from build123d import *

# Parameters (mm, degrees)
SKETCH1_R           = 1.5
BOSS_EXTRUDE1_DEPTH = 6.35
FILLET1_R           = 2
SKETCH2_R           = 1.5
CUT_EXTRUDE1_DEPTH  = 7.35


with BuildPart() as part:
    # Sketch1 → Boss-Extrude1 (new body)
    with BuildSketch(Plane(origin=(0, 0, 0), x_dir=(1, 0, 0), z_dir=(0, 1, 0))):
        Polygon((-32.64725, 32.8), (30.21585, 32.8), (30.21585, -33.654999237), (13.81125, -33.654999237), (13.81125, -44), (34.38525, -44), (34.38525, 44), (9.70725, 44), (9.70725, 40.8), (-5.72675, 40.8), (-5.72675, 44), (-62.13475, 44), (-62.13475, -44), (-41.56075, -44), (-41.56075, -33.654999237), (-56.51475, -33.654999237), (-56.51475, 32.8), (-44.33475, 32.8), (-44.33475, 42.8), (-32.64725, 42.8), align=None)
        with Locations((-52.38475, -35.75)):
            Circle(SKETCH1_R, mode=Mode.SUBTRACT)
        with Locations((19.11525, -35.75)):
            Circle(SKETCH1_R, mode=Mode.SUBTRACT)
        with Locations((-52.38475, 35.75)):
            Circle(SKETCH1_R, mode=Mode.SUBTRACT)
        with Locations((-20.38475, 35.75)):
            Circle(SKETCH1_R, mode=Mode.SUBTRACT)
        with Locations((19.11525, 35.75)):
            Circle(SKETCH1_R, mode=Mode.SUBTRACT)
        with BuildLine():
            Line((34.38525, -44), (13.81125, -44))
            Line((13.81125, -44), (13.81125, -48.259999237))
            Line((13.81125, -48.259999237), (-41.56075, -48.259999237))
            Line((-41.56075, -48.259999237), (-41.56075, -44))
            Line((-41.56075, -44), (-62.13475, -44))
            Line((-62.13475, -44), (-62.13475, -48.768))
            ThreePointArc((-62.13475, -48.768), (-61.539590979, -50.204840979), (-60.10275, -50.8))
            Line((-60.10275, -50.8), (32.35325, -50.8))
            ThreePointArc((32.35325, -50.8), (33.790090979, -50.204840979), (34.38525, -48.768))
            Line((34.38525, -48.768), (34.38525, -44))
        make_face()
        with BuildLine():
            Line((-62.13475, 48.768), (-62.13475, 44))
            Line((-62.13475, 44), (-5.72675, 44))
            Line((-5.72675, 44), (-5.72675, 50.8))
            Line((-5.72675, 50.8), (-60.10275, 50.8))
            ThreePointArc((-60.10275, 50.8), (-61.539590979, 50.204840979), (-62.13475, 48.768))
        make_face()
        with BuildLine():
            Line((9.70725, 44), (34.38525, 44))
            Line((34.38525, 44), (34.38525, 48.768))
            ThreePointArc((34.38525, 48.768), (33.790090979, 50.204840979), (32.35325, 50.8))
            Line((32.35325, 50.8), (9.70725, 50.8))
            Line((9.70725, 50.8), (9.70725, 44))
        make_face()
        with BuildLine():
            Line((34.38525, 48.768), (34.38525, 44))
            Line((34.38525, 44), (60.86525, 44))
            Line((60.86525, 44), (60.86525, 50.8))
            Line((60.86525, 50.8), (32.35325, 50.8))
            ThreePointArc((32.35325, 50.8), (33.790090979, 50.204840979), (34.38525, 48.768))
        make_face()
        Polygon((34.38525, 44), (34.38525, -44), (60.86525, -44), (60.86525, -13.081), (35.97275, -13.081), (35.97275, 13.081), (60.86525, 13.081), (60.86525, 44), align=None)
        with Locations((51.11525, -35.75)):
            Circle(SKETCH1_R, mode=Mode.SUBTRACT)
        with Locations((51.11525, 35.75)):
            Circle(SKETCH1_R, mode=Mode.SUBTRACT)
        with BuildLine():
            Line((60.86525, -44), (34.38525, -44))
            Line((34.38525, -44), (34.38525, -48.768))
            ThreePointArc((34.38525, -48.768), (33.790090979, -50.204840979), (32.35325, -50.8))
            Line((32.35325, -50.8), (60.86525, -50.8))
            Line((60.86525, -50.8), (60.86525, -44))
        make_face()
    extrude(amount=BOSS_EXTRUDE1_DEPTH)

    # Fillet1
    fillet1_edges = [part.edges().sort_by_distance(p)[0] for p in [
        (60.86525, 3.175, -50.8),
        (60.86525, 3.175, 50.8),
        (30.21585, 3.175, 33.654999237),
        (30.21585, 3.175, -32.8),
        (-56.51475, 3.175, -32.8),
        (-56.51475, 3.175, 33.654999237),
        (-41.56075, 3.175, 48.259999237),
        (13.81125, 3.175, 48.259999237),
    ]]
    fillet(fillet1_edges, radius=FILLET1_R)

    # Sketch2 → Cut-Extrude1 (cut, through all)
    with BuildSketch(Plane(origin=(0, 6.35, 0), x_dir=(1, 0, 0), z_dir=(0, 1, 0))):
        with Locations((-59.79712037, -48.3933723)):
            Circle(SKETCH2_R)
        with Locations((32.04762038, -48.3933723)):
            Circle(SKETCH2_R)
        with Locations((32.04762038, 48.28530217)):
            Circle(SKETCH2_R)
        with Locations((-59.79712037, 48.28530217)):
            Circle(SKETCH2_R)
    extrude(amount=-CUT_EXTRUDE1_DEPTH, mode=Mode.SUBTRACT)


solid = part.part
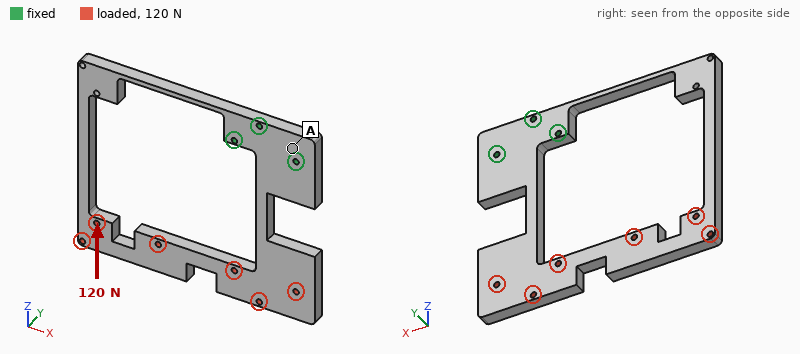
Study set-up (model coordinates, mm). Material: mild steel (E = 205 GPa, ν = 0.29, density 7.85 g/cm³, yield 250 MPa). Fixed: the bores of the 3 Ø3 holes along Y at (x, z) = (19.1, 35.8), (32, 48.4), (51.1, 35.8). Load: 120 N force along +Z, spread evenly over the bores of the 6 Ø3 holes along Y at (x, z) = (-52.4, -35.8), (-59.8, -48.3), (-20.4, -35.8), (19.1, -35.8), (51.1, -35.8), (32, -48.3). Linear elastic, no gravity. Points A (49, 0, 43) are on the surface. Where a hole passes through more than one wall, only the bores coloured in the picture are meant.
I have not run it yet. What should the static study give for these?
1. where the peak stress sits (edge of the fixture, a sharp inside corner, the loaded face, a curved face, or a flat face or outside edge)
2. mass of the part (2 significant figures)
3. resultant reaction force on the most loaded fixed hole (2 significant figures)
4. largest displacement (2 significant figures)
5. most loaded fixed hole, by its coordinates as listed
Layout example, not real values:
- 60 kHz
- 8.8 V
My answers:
- a curved face
- 250 g
- 150 N
- 0.33 mm
- (32, 48.4)
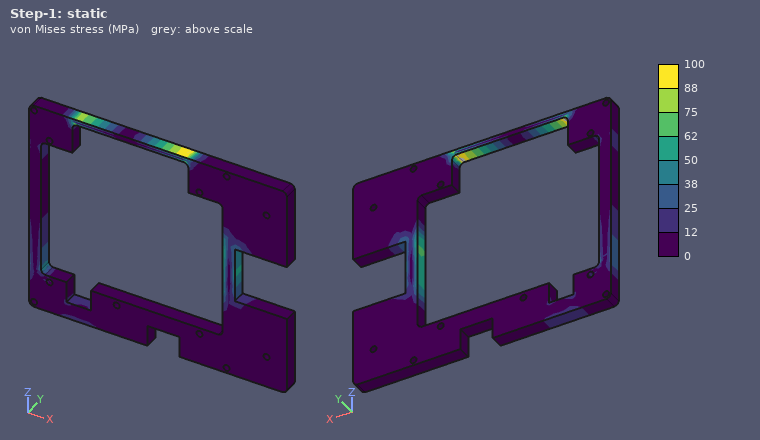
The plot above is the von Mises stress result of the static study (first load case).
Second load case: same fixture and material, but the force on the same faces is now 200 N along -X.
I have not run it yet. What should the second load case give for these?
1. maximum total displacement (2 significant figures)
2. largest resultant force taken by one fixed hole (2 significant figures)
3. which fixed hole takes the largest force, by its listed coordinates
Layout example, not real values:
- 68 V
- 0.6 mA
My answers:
- 0.63 mm
- 610 N
- (51.1, 35.8)
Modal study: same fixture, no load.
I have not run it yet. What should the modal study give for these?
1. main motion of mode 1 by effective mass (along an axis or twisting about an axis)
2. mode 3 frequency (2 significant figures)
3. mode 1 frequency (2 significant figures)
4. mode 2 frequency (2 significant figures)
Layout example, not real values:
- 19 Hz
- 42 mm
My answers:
- along Y
- 350 Hz
- 170 Hz
- 220 Hz
